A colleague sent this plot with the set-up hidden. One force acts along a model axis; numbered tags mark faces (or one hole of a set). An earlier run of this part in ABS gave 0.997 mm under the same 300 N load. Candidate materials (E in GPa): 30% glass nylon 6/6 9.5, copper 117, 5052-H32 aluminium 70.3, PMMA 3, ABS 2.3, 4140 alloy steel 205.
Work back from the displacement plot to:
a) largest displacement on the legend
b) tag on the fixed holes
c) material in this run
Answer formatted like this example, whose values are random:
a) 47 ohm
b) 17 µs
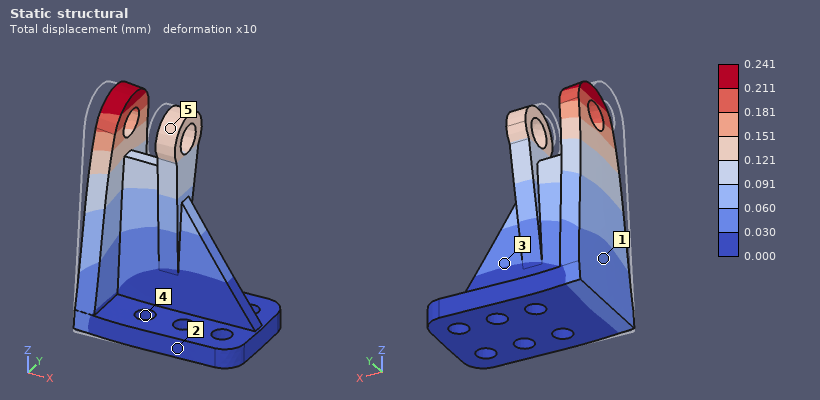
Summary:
a) 0.241 mm
b) 4
c) 30% glass nylon 6/6
